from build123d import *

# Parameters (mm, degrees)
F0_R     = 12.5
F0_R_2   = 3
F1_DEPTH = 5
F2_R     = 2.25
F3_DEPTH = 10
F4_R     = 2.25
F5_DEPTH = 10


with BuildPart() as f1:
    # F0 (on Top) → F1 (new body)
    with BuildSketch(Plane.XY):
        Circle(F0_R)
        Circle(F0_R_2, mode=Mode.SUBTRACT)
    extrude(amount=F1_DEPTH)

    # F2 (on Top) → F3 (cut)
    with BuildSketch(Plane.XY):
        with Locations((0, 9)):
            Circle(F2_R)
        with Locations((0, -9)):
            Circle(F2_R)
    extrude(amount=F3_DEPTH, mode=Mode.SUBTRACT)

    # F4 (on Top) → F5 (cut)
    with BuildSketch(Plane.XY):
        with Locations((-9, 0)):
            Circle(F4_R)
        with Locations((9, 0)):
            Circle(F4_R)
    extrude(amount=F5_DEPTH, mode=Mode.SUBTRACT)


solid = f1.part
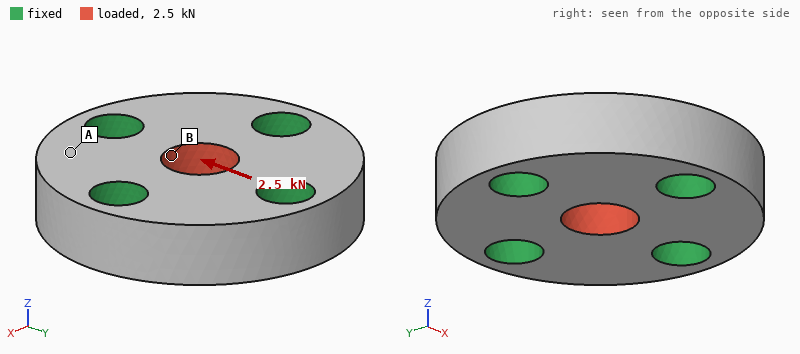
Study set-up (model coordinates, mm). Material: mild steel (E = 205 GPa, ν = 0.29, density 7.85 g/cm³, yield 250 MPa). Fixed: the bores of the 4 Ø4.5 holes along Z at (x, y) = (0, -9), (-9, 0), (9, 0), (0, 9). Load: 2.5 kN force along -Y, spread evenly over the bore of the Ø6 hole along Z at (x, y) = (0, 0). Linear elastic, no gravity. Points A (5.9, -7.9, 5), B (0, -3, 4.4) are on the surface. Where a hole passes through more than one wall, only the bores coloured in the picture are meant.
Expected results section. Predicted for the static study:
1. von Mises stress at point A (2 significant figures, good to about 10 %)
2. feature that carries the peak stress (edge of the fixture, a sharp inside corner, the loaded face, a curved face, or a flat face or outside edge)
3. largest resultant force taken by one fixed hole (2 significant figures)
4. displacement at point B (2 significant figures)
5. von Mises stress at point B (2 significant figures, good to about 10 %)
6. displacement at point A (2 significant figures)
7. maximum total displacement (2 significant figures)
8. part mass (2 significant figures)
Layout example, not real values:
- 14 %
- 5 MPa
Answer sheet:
- 4.9 MPa
- the loaded face
- 840 N
- 0.56 µm
- 29 MPa
- 0.21 µm
- 0.75 µm
- 16 g
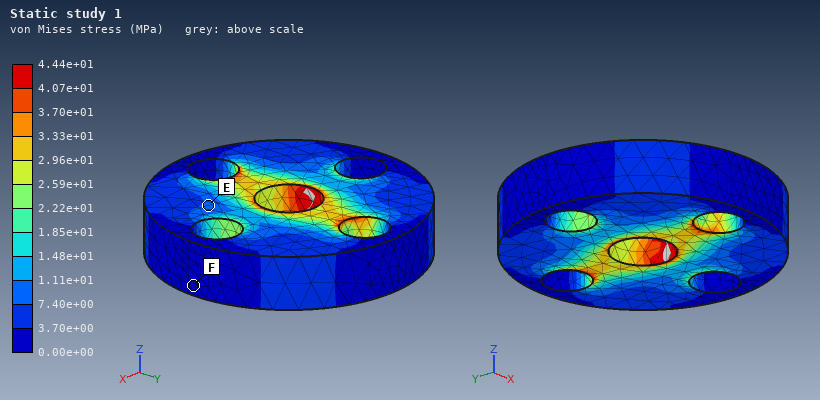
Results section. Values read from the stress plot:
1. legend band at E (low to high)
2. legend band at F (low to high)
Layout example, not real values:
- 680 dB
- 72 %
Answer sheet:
- 7.40e+00 to 1.11e+01 MPa
- 0.00e+00 to 3.70e+00 MPa
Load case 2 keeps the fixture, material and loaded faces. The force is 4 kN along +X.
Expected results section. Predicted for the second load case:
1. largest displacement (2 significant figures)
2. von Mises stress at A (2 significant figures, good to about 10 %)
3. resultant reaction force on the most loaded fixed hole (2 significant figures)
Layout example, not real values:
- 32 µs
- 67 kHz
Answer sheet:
- 1.2 µm
- 8.3 MPa
- 1.3 kN
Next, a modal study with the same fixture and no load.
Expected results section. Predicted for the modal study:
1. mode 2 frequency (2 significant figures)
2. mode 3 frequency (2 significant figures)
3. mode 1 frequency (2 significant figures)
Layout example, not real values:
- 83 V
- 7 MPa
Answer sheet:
- 100 kHz
- 100 kHz
- 99 kHz
